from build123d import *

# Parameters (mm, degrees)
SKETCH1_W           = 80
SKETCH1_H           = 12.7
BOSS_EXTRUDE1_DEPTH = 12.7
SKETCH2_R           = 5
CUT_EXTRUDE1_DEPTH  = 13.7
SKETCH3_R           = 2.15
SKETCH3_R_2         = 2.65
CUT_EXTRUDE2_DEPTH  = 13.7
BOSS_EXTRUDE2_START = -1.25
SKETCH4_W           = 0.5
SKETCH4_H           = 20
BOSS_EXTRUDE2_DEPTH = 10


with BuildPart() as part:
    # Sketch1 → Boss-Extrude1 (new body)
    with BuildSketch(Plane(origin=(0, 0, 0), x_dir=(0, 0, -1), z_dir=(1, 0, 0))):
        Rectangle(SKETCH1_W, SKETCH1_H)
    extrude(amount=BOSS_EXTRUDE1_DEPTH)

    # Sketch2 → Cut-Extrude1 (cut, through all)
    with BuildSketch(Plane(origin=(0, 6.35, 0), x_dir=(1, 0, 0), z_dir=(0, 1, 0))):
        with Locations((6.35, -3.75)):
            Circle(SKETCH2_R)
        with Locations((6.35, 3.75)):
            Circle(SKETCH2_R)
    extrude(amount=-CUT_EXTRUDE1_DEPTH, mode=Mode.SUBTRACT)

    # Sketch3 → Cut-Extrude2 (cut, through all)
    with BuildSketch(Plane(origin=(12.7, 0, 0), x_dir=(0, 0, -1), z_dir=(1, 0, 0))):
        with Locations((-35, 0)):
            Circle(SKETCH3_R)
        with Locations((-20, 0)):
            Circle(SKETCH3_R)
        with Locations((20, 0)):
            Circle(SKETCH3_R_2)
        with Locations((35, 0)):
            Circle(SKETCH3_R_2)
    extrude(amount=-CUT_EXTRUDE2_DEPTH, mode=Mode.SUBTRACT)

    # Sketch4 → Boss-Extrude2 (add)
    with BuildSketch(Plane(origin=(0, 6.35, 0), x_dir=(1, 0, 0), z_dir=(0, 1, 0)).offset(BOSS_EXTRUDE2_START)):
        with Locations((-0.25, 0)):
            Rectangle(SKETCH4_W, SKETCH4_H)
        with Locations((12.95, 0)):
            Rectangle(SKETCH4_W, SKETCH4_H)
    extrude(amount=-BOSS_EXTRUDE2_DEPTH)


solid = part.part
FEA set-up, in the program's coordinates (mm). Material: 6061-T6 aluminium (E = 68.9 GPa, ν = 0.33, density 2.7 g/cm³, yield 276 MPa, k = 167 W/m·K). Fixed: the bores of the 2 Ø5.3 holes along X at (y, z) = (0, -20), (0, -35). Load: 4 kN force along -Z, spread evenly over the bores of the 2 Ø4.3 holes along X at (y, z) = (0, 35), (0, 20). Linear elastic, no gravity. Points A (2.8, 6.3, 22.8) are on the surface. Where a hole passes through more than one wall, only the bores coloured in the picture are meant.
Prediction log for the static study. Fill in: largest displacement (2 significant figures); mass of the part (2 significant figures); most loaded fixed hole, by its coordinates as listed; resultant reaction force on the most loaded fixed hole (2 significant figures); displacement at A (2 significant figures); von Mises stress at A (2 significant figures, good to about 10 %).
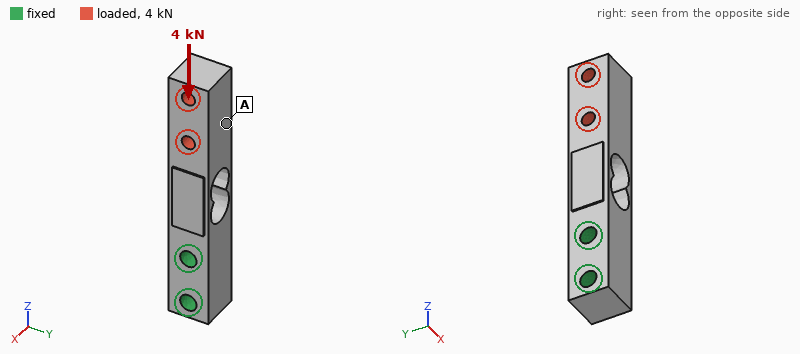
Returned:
40 µm
28 g
(0, -20)
3.7 kN
35 µm
22 MPa
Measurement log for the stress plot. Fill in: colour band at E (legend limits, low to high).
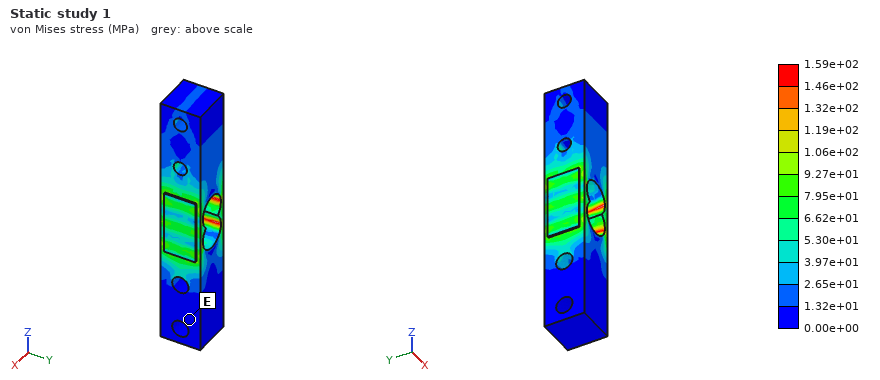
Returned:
0.00e+00 to 1.32e+01 MPa
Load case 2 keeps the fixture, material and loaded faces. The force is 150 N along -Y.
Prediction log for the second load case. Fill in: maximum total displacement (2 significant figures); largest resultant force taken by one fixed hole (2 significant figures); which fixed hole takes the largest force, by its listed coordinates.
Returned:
0.12 mm
300 N
(0, -20)
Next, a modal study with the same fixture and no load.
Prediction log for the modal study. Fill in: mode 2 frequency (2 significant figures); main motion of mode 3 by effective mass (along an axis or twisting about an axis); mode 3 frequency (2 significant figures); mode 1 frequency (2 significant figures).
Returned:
2000 Hz
twisting about Z
7800 Hz
2000 Hz
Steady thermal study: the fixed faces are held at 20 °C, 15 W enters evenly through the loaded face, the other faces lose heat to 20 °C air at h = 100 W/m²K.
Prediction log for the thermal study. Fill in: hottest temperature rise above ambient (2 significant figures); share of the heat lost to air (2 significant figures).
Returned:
30 K
42 %
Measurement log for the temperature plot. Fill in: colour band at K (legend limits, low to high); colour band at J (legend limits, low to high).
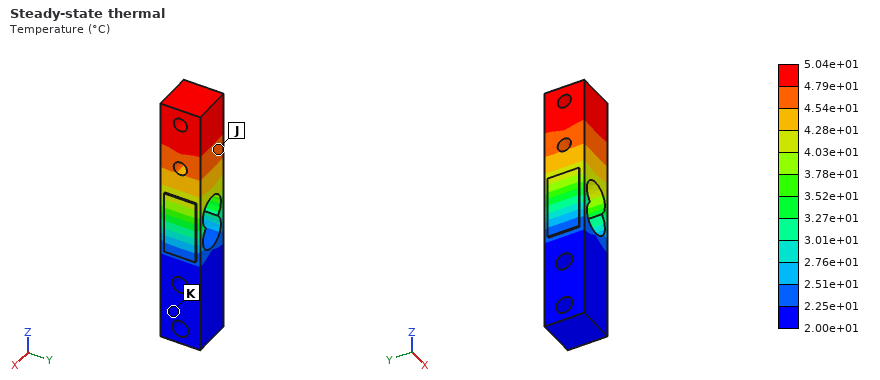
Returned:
2.00e+01 to 2.25e+01 °C
4.54e+01 to 4.79e+01 °C
